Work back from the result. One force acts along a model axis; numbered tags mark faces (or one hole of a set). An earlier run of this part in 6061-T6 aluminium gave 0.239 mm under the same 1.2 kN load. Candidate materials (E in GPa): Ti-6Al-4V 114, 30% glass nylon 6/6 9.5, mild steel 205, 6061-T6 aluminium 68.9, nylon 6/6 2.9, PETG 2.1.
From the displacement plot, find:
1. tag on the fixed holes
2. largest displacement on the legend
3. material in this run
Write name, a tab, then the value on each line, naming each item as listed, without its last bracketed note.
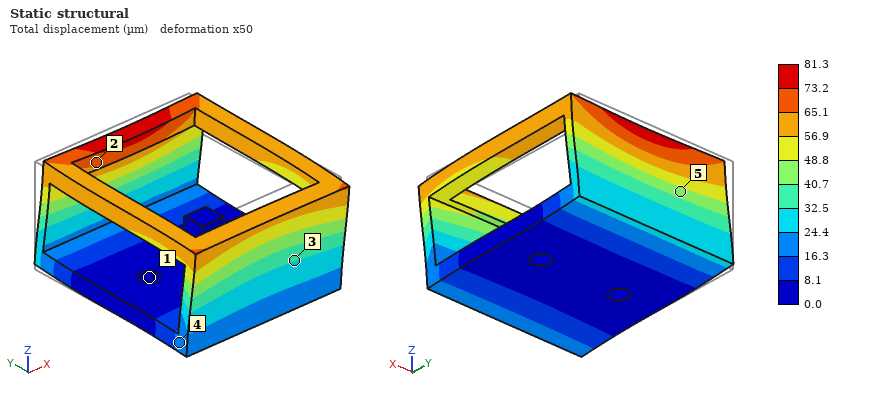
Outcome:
tag on the fixed holes	1
largest displacement on the legend	81.3 µm
material in this run	mild steel
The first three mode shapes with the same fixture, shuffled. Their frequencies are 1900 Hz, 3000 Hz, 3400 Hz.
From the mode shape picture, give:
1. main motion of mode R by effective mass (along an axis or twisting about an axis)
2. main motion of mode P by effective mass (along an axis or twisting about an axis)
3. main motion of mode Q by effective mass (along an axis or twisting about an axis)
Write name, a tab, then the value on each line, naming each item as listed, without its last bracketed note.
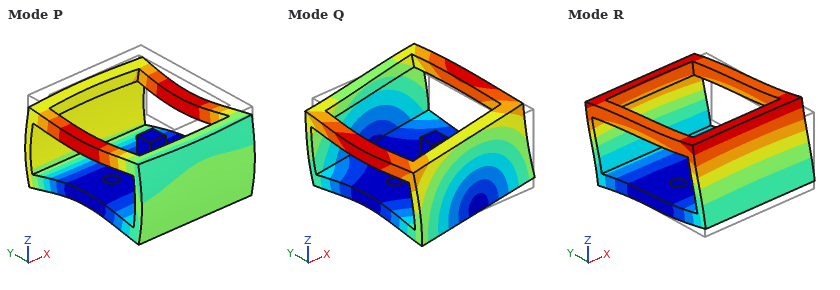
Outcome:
main motion of mode R by effective mass	along Y
main motion of mode P by effective mass	along Z
main motion of mode Q by effective mass	along X
